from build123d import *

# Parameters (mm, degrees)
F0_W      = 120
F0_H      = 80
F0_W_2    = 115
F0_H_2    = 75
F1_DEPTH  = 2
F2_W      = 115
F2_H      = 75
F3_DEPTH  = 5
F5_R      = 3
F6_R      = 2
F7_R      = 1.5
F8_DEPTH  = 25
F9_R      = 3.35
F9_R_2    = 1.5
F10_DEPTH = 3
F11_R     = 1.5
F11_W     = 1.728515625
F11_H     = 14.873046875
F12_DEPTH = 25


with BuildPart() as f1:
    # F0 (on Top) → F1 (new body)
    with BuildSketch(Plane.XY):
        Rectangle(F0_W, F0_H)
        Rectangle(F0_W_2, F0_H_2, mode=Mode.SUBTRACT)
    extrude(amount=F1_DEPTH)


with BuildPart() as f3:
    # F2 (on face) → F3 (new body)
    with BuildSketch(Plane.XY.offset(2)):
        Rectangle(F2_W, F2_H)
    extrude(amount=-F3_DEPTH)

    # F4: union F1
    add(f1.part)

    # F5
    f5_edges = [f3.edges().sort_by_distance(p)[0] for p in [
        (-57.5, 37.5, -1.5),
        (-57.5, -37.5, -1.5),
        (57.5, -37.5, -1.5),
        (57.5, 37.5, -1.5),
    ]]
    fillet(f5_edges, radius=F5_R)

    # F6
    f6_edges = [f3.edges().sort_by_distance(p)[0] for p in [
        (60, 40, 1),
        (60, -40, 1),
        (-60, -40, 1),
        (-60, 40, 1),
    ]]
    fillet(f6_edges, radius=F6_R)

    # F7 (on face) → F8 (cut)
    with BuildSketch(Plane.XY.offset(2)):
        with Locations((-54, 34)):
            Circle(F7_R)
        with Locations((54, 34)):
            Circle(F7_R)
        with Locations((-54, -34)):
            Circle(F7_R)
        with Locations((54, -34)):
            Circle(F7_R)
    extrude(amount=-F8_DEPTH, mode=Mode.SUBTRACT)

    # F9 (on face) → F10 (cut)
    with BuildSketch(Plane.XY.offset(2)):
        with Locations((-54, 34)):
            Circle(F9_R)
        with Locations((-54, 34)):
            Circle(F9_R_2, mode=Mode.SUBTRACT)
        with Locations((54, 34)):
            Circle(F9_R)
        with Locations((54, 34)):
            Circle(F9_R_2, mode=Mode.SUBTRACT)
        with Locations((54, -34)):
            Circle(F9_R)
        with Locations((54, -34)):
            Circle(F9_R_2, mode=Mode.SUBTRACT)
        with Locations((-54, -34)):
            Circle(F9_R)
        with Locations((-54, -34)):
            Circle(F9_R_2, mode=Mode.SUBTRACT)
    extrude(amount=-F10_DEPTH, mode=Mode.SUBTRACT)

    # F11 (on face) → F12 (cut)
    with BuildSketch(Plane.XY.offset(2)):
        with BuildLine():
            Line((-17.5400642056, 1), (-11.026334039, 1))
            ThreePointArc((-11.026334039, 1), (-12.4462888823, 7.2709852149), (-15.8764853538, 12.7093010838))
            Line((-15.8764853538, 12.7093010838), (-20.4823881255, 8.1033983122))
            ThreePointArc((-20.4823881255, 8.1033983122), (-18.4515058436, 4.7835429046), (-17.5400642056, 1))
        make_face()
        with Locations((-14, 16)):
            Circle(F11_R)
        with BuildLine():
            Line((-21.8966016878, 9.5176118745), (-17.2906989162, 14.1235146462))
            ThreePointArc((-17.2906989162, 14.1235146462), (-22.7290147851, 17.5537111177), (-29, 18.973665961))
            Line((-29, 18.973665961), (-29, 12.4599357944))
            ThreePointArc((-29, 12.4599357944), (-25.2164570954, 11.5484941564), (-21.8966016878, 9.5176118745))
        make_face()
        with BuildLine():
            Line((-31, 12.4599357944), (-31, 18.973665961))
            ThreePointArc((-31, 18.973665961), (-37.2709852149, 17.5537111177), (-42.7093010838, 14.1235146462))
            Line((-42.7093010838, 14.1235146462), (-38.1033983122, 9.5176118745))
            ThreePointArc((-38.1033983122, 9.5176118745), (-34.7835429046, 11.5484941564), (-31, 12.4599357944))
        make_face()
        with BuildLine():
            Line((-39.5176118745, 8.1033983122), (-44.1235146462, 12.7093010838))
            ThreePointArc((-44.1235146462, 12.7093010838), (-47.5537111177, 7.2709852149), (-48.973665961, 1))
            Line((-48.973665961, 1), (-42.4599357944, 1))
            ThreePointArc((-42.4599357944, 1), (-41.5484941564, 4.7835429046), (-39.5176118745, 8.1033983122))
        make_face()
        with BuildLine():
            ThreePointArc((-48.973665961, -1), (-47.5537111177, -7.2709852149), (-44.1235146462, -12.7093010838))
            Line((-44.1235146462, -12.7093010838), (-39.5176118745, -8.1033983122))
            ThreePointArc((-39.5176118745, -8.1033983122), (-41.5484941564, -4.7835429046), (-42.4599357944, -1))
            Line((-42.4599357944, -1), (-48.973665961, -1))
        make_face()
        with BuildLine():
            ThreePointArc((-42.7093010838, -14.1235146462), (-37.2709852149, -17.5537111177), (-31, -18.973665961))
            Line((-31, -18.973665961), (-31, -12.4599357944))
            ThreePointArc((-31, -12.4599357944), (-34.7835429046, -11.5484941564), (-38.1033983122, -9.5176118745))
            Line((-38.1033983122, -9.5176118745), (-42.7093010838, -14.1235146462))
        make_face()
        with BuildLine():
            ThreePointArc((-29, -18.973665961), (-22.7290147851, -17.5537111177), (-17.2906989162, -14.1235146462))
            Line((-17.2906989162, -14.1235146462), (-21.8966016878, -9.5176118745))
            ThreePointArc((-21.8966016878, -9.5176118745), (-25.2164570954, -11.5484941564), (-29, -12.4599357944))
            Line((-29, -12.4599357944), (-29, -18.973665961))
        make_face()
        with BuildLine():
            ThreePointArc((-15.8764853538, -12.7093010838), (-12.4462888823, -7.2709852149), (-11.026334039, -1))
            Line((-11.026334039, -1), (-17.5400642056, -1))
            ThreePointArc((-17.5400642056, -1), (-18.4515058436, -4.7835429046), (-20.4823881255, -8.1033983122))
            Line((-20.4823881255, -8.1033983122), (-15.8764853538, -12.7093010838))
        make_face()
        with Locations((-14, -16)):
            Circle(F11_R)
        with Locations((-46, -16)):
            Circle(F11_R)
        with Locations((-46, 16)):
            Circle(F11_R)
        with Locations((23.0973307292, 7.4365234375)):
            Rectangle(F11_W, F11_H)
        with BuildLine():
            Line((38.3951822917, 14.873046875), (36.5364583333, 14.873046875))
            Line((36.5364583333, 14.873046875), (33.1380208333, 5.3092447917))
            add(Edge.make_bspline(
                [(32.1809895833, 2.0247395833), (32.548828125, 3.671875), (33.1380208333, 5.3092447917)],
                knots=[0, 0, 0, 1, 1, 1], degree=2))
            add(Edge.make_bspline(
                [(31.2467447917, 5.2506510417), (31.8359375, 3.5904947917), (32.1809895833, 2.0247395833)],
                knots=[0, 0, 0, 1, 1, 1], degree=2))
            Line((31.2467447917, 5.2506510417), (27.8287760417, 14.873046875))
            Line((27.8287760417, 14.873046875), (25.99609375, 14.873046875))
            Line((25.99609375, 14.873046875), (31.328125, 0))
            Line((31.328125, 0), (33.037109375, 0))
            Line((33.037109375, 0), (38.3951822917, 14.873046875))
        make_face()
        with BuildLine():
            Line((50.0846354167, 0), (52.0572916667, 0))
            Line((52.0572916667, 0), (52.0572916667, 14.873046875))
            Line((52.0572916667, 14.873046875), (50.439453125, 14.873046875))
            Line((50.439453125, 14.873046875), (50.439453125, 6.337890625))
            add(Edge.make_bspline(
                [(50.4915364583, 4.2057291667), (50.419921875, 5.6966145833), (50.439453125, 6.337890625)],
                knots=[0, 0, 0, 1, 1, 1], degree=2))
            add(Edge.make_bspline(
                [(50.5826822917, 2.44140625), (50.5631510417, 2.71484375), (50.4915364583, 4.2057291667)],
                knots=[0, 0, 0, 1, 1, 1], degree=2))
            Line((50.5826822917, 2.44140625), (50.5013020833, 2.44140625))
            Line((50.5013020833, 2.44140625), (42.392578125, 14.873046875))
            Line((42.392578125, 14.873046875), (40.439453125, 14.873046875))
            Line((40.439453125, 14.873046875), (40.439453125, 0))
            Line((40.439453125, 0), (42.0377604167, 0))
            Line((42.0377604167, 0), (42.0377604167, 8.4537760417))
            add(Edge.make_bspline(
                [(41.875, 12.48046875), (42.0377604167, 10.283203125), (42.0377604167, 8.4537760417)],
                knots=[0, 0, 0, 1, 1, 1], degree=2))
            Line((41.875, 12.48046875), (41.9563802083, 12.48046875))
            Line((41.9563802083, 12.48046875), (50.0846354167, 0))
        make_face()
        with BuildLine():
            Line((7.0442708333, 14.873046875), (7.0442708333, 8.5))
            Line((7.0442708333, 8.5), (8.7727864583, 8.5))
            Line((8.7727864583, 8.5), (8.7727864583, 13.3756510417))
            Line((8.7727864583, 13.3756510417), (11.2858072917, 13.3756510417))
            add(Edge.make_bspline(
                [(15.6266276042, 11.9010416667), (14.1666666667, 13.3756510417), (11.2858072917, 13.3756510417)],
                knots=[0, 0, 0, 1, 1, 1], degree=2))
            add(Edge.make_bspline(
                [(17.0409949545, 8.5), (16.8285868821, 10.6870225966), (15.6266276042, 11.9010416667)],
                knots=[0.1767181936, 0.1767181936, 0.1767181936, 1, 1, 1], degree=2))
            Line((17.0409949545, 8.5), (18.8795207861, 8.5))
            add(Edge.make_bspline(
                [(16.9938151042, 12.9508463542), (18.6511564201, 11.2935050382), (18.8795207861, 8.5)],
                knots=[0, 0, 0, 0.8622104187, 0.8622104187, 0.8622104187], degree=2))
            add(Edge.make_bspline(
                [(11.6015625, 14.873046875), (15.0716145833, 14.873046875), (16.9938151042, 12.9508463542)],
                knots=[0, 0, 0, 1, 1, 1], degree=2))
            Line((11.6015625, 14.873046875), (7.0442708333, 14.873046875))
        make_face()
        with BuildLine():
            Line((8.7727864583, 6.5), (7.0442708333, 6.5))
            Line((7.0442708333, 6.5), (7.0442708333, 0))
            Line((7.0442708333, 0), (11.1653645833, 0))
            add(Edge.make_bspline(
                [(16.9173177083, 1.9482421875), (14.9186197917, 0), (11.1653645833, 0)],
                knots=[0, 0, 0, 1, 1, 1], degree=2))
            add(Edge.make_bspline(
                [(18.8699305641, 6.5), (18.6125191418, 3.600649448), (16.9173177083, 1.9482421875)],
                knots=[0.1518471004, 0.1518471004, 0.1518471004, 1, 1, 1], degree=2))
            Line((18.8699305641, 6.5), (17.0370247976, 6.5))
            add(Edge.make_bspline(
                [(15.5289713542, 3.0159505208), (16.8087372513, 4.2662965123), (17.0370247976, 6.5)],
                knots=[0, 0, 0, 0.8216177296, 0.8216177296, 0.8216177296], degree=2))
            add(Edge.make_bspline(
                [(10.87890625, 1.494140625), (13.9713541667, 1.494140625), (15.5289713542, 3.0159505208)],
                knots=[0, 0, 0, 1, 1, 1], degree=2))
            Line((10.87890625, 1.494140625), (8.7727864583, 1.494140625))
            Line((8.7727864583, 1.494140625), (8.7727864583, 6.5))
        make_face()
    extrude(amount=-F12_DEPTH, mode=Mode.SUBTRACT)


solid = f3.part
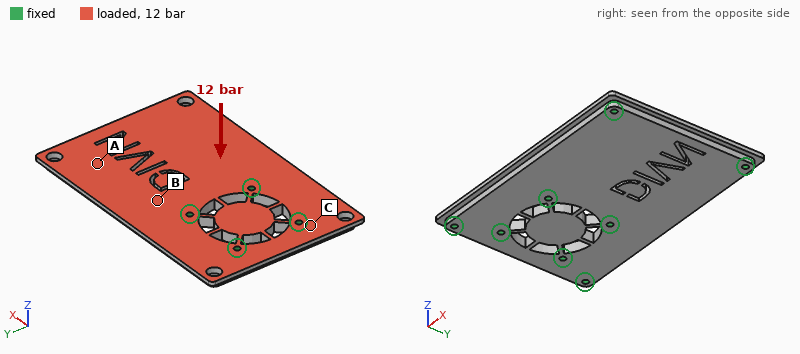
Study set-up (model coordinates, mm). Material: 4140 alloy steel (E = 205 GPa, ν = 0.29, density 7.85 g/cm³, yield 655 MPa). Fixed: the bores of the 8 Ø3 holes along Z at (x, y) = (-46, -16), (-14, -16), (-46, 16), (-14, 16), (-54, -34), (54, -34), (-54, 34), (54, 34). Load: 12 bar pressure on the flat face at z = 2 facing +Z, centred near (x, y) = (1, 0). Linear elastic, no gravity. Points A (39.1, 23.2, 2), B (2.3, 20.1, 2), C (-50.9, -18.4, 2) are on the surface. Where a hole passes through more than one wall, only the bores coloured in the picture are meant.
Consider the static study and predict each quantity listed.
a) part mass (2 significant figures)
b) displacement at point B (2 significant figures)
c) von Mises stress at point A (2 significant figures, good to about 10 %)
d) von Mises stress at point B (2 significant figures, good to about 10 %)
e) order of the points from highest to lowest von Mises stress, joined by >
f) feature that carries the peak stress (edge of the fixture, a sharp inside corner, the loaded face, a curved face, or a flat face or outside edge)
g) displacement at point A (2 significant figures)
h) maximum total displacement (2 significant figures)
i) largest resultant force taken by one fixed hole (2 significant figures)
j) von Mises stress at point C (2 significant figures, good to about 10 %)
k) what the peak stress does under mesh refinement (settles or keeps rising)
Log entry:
320 g
0.047 mm
93 MPa
54 MPa
A > B > C
edge of the fixture
0.075 mm
0.14 mm
2.8 kN
25 MPa
keeps rising
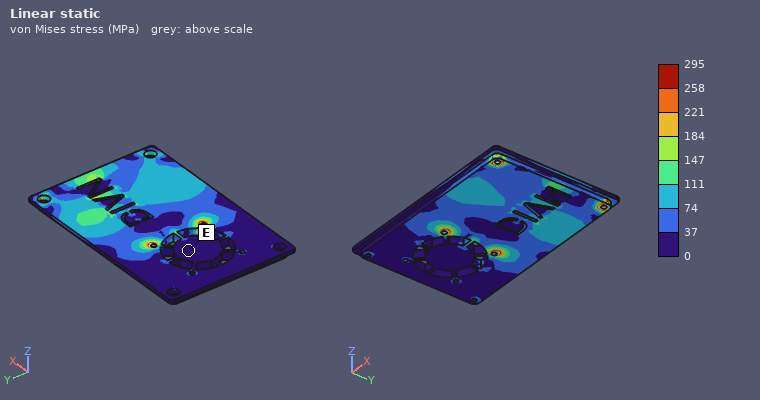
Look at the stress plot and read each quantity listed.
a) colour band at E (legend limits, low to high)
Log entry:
0 to 37 MPa
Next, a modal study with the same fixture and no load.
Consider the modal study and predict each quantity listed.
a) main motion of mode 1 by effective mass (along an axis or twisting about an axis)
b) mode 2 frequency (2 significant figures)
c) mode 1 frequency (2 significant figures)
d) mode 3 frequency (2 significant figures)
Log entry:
along Z
4400 Hz
3200 Hz
4500 Hz
